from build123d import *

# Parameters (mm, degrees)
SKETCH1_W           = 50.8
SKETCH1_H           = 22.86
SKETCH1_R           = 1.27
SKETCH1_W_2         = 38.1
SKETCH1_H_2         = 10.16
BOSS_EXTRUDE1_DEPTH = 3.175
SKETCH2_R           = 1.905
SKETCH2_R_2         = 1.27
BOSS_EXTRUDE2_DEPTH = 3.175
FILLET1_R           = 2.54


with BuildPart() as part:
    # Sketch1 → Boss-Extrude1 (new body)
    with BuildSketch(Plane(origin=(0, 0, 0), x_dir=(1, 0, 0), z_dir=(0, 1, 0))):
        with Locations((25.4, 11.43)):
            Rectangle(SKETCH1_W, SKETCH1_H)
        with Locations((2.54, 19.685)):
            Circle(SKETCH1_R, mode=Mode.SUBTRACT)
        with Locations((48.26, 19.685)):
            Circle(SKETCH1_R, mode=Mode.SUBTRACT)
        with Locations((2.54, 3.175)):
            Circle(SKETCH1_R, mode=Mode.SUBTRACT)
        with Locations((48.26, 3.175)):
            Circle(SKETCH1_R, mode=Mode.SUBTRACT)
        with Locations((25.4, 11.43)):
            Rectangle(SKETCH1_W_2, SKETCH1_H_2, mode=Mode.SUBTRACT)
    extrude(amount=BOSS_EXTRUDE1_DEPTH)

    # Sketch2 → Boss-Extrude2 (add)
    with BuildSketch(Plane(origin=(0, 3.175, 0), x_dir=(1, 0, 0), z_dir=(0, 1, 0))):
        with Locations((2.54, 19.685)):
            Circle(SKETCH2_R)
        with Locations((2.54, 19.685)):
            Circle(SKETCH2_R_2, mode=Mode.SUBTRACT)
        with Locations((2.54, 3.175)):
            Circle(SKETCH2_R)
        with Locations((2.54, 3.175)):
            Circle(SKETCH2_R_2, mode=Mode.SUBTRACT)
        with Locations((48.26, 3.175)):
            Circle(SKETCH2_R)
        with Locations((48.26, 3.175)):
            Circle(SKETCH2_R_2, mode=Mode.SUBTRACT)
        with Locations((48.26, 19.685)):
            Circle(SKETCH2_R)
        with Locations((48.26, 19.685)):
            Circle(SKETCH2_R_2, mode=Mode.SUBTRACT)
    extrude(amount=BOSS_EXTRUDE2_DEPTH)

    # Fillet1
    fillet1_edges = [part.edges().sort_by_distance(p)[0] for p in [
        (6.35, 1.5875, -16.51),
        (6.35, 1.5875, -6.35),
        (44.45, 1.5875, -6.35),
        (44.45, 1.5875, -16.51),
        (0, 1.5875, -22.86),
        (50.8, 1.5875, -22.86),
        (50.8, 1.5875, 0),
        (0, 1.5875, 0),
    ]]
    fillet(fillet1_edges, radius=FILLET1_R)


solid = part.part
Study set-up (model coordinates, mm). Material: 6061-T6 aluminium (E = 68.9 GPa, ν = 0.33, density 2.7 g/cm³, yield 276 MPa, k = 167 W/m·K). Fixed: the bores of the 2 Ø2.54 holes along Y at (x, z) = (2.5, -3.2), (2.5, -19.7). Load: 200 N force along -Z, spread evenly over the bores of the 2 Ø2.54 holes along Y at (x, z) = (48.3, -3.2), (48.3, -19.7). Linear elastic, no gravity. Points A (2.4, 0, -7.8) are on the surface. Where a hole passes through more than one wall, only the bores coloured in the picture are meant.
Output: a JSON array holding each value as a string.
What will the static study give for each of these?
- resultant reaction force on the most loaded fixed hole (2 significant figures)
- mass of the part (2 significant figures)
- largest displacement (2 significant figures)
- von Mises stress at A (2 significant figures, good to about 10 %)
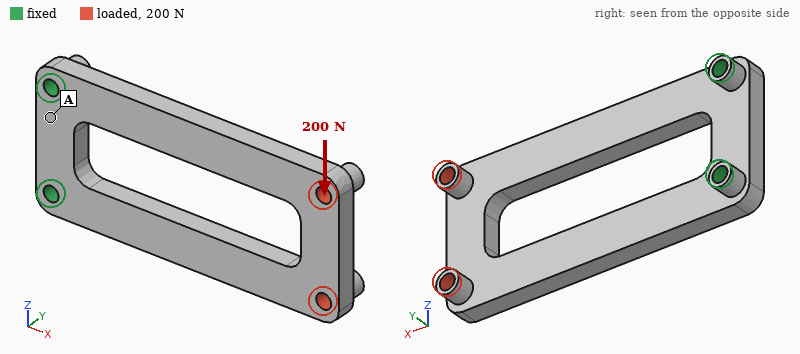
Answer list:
["450 N", "6.7 g", "0.21 mm", "17 MPa"]
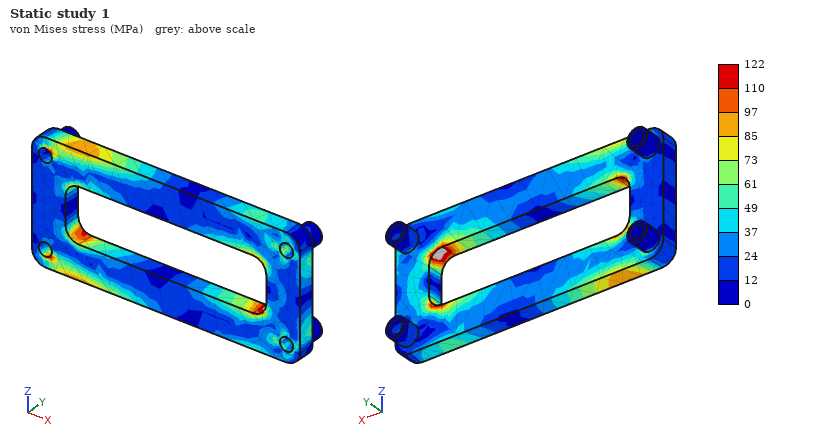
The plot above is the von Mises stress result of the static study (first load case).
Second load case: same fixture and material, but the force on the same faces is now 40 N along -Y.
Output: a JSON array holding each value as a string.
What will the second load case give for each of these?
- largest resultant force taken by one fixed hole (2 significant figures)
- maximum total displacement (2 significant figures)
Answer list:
["20 N", "0.55 mm"]
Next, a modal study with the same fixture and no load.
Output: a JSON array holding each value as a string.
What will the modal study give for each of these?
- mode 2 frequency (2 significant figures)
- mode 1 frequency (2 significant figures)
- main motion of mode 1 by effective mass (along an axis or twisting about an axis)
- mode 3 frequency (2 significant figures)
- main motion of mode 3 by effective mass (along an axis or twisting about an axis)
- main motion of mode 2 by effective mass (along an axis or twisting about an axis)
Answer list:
["3300 Hz", "1000 Hz", "along Y", "3500 Hz", "twisting about X", "along Z"]
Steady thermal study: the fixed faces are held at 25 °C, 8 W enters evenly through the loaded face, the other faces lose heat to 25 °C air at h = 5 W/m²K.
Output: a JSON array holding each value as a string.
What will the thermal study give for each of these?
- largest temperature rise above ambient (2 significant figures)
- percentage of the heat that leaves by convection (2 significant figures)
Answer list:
["55 K", "3.8 %"]
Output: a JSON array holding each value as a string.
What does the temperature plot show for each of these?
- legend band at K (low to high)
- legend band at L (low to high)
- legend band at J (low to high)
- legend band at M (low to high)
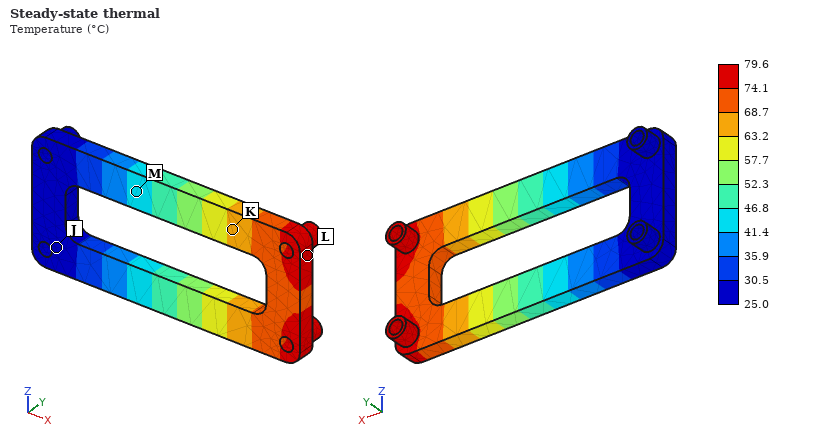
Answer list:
["63.2 to 68.7 °C", "74.1 to 79.6 °C", "25.0 to 30.5 °C", "41.4 to 46.8 °C"]
